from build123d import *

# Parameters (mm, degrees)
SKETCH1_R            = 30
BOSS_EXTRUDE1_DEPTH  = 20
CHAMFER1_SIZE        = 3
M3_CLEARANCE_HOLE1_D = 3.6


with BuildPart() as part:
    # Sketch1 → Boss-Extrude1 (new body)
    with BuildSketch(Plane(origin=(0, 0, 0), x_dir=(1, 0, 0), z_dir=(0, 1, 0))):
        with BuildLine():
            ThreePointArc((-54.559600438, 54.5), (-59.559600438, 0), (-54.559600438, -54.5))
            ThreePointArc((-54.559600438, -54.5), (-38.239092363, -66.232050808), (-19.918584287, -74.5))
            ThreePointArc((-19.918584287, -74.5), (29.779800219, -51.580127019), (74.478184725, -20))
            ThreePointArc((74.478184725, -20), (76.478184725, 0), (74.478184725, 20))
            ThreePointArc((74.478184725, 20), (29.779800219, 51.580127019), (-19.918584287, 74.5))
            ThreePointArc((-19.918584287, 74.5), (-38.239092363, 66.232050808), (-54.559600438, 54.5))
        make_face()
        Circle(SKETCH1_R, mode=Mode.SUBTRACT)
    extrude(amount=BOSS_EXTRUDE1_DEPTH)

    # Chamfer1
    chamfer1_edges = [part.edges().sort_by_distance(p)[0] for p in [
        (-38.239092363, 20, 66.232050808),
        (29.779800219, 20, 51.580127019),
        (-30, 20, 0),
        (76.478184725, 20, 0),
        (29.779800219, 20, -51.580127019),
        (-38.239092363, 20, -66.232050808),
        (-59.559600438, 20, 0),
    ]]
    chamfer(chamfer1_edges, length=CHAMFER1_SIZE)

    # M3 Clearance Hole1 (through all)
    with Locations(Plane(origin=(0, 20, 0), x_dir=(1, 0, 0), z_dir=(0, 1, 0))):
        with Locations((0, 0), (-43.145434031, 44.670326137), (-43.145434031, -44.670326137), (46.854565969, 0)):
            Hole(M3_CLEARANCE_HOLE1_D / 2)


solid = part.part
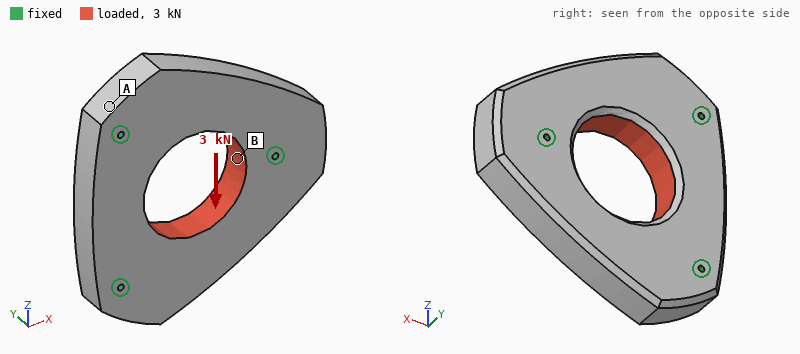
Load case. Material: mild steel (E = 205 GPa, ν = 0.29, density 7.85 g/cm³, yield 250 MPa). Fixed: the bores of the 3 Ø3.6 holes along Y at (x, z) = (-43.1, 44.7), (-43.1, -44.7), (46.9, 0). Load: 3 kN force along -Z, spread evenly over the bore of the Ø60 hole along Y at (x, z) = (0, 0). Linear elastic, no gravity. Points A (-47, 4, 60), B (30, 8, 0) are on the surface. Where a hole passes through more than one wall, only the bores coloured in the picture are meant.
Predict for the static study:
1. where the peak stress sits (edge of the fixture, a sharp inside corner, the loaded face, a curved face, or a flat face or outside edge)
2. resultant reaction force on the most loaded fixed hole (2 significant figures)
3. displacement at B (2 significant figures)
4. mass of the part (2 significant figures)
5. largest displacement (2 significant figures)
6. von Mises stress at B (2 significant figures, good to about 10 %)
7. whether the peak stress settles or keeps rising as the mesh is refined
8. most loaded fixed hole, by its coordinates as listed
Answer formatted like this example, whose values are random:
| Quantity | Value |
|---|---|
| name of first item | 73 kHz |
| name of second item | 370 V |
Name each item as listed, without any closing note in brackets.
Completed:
| Quantity | Value |
|---|---|
| where the peak stress sits | edge of the fixture |
| resultant reaction force on the most loaded fixed hole | 1.5 kN |
| displacement at B | 0.42 µm |
| mass of the part | 1.8 kg |
| largest displacement | 0.68 µm |
| von Mises stress at B | 1.6 MPa |
| whether the peak stress settles or keeps rising as the mesh is refined | keeps rising |
| most loaded fixed hole, by its coordinates as listed | (46.9, 0) |
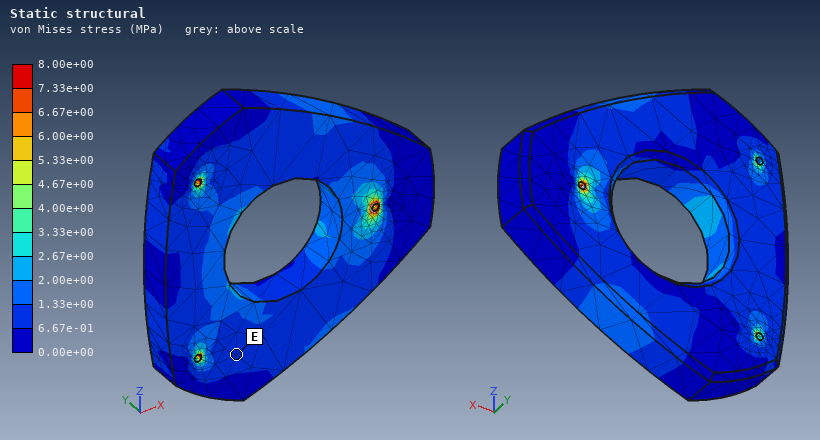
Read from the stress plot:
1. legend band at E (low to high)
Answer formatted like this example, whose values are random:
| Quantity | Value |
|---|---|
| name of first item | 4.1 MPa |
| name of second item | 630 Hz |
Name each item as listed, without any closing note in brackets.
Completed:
| Quantity | Value |
|---|---|
| legend band at E | 6.67e-01 to 1.33e+00 MPa |
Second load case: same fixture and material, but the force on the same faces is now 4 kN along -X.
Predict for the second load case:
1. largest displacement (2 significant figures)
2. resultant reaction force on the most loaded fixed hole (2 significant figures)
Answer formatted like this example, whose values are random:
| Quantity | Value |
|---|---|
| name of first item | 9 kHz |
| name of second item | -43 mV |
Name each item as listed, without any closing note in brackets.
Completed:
| Quantity | Value |
|---|---|
| largest displacement | 1.0 µm |
| resultant reaction force on the most loaded fixed hole | 1.4 kN |
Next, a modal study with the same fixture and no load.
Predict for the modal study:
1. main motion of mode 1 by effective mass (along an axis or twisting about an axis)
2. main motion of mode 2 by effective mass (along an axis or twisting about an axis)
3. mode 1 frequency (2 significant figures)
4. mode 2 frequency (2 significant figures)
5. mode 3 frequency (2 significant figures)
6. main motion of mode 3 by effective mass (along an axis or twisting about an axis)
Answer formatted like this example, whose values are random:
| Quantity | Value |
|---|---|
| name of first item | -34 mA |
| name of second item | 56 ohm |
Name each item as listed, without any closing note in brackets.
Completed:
| Quantity | Value |
|---|---|
| main motion of mode 1 by effective mass | twisting about X |
| main motion of mode 2 by effective mass | along Y |
| mode 1 frequency | 4600 Hz |
| mode 2 frequency | 5300 Hz |
| mode 3 frequency | 8100 Hz |
| main motion of mode 3 by effective mass | along Y |
